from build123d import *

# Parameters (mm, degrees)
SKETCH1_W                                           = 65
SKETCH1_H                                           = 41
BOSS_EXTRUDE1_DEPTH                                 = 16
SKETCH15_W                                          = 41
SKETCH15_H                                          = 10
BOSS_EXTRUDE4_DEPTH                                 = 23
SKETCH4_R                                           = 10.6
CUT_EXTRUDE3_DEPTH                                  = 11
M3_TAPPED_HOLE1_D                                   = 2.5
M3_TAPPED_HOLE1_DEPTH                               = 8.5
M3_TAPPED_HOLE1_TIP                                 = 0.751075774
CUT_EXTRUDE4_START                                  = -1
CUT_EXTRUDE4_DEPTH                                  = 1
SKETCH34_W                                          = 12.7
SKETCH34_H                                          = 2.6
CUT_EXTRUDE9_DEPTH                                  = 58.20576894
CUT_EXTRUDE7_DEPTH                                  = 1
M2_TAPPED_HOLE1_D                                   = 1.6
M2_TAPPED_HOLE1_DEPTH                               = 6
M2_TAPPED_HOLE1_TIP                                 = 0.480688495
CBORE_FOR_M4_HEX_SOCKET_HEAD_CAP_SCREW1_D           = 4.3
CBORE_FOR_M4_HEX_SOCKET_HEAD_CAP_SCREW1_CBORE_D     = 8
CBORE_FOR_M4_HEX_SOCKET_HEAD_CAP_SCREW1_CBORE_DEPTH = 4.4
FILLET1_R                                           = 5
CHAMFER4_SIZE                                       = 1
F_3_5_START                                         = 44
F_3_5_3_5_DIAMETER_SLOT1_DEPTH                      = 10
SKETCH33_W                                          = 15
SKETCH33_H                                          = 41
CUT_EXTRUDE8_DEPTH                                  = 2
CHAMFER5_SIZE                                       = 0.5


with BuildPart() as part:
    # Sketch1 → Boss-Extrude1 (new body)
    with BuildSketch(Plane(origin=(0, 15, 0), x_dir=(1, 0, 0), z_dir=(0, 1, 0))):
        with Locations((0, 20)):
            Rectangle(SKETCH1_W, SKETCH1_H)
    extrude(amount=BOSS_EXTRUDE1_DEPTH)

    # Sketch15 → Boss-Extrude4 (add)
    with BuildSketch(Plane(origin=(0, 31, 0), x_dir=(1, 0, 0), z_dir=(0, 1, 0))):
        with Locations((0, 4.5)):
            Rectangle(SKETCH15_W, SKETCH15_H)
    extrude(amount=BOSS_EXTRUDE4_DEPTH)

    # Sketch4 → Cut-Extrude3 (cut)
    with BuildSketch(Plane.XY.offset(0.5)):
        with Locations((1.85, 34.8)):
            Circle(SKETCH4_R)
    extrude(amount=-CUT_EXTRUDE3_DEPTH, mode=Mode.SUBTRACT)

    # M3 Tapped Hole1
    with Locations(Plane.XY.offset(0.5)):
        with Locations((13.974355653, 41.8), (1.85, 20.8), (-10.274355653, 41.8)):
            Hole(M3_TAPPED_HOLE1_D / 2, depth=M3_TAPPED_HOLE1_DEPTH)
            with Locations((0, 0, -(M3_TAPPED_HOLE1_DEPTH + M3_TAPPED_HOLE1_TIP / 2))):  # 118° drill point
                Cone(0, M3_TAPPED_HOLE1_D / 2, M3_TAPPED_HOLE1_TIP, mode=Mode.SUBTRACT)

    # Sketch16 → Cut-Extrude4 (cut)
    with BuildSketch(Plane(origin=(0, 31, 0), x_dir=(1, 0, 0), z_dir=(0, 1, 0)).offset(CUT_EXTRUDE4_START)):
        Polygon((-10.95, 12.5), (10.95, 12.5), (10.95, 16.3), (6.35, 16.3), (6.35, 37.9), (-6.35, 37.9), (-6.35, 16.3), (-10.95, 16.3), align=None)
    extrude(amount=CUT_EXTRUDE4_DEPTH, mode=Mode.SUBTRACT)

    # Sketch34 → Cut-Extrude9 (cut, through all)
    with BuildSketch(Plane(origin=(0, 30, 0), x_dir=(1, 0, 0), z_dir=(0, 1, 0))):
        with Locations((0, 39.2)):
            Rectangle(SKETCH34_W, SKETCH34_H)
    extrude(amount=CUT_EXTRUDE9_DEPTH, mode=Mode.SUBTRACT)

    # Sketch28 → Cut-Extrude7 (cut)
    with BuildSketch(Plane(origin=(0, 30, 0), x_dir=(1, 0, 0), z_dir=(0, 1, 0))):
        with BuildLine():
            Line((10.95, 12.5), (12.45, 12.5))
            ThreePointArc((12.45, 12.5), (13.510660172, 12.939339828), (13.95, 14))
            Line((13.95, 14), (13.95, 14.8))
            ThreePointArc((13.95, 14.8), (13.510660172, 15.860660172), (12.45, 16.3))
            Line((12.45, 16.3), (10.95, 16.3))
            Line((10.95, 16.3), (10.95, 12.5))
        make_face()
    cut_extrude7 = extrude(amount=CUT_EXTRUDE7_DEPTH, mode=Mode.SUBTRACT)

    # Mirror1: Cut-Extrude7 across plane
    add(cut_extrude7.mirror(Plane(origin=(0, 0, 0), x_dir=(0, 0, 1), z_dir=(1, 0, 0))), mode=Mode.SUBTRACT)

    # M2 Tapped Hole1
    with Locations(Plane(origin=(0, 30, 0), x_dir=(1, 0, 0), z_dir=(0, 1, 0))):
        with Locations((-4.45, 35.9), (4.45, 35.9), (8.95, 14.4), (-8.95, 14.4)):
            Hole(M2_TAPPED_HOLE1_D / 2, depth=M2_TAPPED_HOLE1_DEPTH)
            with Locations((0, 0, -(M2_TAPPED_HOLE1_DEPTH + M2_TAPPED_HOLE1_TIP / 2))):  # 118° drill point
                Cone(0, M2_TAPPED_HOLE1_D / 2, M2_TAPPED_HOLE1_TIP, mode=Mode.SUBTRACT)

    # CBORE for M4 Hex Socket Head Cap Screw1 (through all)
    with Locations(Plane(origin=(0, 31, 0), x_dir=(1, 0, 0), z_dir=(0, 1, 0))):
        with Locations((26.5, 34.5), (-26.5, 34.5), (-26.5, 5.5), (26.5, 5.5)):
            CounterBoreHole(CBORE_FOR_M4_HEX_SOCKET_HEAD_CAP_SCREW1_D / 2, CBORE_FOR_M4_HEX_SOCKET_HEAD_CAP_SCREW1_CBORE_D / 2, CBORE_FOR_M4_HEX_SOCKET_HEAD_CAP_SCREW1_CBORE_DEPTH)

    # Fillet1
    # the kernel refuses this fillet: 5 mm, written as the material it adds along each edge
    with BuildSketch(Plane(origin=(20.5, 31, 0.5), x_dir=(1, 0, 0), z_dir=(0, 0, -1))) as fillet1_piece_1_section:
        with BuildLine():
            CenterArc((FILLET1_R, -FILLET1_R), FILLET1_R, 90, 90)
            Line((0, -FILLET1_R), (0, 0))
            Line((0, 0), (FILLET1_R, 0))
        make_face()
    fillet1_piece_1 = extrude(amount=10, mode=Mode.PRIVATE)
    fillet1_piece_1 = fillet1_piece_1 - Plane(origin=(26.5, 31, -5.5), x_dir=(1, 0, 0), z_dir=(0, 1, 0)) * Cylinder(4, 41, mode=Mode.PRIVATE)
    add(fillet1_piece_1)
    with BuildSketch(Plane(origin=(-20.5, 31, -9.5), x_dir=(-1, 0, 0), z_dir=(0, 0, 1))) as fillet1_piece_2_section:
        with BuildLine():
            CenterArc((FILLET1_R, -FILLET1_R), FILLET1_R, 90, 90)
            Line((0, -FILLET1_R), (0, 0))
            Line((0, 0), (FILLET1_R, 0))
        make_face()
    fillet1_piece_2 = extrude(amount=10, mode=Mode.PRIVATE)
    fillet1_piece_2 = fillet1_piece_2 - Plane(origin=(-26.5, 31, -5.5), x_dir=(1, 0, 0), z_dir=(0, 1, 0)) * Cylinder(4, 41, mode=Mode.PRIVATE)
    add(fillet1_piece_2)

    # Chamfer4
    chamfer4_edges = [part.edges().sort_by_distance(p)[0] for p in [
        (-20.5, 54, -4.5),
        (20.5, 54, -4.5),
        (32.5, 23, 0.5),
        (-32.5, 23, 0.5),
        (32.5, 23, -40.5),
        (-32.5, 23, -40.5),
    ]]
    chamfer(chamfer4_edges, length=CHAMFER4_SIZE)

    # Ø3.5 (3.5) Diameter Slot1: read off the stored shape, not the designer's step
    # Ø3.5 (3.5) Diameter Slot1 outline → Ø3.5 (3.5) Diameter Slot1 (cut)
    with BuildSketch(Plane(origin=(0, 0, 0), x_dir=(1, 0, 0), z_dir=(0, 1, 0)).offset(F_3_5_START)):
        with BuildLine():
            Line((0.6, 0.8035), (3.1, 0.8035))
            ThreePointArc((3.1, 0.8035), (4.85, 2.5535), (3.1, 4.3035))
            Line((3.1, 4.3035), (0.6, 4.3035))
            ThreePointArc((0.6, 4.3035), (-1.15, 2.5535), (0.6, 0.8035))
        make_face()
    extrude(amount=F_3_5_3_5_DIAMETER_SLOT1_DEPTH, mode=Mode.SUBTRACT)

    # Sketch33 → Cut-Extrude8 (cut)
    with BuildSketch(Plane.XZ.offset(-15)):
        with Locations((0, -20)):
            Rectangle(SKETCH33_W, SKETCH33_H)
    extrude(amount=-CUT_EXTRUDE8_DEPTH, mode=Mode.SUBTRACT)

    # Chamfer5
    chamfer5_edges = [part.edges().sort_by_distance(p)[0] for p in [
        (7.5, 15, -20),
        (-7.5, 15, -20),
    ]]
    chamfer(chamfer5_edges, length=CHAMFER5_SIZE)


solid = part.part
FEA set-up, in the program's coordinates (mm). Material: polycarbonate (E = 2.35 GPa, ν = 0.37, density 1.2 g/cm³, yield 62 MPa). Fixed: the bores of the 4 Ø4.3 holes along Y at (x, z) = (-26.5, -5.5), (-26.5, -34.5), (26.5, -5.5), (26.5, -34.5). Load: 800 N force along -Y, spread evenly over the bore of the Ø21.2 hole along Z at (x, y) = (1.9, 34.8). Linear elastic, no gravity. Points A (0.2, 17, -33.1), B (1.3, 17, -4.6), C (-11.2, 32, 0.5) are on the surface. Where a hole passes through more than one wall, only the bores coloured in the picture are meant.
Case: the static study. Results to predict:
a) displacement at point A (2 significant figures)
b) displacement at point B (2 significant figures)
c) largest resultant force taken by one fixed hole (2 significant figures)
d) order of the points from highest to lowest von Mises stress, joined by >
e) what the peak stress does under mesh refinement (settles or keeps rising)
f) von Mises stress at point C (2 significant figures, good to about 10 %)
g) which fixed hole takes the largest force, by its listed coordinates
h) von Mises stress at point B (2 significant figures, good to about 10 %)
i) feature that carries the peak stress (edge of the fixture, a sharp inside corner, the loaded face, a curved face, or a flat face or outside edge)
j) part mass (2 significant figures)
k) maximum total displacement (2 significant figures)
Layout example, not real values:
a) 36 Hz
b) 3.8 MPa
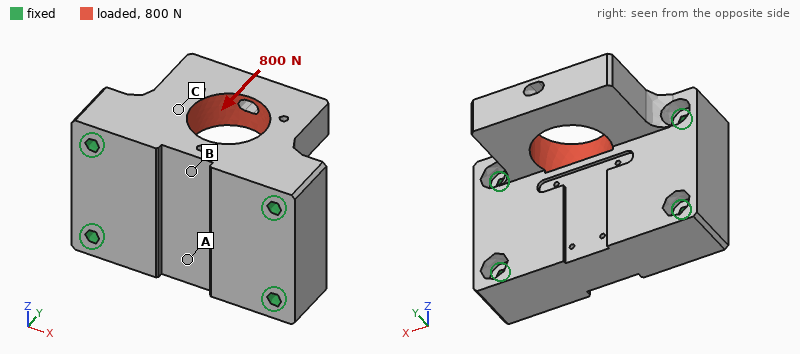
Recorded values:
a) 14 µm
b) 65 µm
c) 440 N
d) B > C > A
e) keeps rising
f) 1.7 MPa
g) (26.5, -5.5)
h) 3.0 MPa
i) edge of the fixture
j) 54 g
k) 81 µm
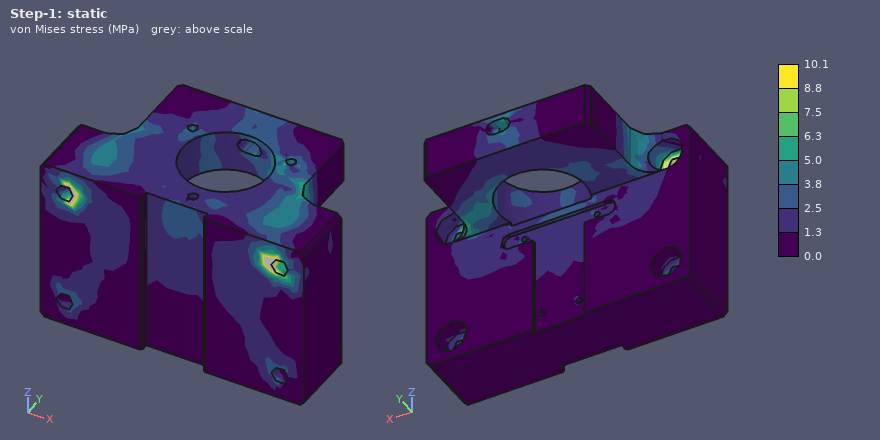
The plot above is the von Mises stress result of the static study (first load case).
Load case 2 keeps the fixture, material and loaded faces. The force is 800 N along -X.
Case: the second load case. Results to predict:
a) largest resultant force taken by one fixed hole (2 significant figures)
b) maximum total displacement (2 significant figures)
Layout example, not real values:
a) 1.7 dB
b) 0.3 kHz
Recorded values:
a) 360 N
b) 95 µm
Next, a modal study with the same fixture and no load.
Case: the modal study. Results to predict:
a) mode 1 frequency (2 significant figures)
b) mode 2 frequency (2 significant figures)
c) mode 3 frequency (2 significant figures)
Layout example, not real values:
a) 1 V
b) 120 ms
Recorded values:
a) 2100 Hz
b) 3600 Hz
c) 4000 Hz
